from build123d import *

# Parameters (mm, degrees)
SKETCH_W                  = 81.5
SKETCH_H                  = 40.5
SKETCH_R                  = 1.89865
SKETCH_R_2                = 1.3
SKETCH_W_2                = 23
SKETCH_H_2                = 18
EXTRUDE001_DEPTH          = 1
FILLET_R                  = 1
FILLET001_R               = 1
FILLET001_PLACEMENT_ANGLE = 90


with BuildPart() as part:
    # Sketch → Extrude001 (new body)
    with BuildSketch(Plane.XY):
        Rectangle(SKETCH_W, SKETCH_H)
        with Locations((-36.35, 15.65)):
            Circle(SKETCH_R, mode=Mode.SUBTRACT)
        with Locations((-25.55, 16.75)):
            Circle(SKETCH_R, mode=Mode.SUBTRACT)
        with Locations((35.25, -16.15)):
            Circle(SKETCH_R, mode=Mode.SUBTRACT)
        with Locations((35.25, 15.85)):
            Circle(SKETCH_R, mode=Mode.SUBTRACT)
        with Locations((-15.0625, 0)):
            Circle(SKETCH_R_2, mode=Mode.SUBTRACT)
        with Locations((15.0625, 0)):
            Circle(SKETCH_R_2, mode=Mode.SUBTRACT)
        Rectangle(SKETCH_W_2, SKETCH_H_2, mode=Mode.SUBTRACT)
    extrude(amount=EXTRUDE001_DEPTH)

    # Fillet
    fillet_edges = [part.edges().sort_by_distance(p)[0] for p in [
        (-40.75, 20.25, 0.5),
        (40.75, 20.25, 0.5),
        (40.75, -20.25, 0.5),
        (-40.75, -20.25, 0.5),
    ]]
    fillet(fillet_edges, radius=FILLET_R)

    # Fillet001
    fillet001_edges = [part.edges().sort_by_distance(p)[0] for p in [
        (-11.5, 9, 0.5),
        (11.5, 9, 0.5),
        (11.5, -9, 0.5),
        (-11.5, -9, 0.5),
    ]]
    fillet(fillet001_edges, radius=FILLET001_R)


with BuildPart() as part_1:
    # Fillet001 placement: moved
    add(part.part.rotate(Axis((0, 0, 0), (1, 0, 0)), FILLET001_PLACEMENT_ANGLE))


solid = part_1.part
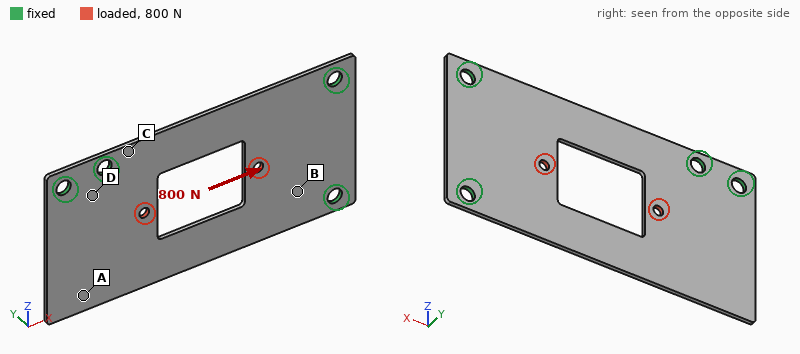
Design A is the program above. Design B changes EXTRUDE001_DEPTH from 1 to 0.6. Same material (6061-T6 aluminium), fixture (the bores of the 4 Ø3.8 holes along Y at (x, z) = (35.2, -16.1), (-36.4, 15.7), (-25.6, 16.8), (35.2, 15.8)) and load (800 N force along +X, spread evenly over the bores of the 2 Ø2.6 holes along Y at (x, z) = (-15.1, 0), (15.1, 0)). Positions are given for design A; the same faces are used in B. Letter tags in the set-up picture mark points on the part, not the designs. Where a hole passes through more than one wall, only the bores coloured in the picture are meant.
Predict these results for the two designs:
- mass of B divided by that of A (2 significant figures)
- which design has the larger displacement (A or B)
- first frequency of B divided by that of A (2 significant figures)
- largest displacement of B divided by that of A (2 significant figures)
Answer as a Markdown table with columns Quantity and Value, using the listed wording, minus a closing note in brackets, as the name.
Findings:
| Quantity | Value |
|---|---|
| mass of B divided by that of A | 0.60 |
| which design has the larger displacement | B |
| first frequency of B divided by that of A | 0.60 |
| largest displacement of B divided by that of A | 1.7 |
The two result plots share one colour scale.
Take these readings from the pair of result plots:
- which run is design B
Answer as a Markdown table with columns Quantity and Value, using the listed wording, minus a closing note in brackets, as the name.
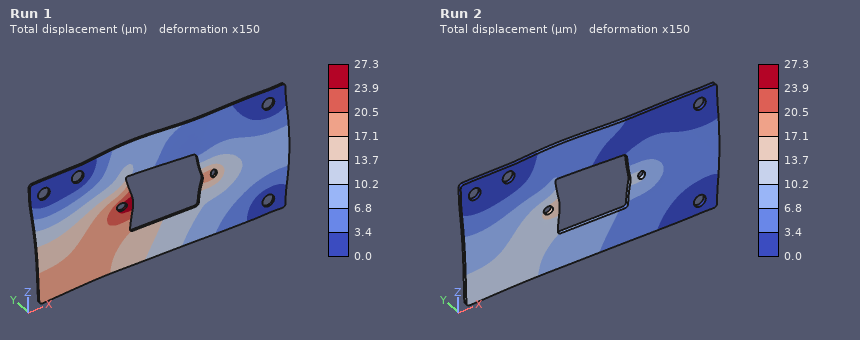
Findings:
| Quantity | Value |
|---|---|
| which run is design B | Run 1 |
